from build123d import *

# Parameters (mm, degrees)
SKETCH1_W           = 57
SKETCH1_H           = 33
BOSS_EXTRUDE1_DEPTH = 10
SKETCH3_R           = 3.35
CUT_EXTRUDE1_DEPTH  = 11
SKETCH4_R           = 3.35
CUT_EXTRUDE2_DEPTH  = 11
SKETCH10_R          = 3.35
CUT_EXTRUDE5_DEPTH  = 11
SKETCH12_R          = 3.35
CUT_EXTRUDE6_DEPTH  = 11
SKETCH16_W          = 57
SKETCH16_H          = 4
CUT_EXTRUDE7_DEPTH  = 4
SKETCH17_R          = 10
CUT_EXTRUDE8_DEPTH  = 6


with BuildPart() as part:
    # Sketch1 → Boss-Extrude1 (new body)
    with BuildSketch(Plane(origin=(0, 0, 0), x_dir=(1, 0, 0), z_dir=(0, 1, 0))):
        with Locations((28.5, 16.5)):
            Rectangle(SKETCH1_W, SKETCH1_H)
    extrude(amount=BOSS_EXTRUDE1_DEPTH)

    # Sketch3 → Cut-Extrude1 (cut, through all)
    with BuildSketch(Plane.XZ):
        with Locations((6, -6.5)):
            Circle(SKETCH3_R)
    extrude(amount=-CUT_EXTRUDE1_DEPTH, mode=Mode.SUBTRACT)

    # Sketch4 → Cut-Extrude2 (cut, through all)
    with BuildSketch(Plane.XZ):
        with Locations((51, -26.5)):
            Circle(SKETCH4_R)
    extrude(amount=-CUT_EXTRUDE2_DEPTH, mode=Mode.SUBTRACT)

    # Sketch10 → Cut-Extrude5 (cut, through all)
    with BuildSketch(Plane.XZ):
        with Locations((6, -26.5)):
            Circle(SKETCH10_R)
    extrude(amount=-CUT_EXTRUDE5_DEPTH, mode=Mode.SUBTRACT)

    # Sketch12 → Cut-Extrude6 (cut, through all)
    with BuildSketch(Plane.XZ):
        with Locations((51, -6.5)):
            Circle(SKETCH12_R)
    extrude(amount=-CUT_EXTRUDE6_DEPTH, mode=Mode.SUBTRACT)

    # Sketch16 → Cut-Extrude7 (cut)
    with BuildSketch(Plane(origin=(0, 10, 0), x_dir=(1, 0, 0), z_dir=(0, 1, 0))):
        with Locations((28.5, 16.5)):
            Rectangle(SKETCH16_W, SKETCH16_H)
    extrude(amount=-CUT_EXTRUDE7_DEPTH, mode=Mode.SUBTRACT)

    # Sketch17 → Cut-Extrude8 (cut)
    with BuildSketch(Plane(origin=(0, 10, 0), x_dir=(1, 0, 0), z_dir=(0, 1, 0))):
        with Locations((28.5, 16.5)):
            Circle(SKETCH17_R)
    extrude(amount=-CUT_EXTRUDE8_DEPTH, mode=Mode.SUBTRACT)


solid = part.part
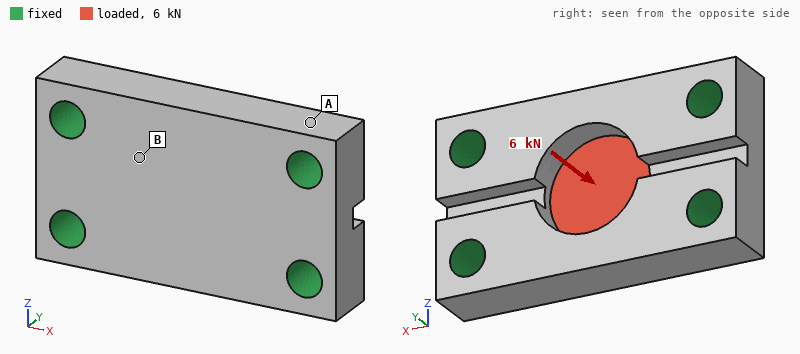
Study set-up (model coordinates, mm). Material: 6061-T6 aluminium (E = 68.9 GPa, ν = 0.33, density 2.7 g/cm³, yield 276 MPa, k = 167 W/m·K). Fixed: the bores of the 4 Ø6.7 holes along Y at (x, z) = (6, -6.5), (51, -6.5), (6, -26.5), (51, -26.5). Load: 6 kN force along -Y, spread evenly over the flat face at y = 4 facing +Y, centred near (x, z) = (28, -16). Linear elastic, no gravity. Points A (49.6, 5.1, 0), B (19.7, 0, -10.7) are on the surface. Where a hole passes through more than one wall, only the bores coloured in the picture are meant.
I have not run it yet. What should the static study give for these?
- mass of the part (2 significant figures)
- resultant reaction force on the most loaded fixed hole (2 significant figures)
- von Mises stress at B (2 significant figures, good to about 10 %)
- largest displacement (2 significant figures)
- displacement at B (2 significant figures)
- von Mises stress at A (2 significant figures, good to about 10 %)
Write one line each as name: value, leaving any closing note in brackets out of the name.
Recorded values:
mass of the part: 40 g
resultant reaction force on the most loaded fixed hole: 1.6 kN
von Mises stress at B: 36 MPa
largest displacement: 40 µm
displacement at B: 18 µm
von Mises stress at A: 14 MPa
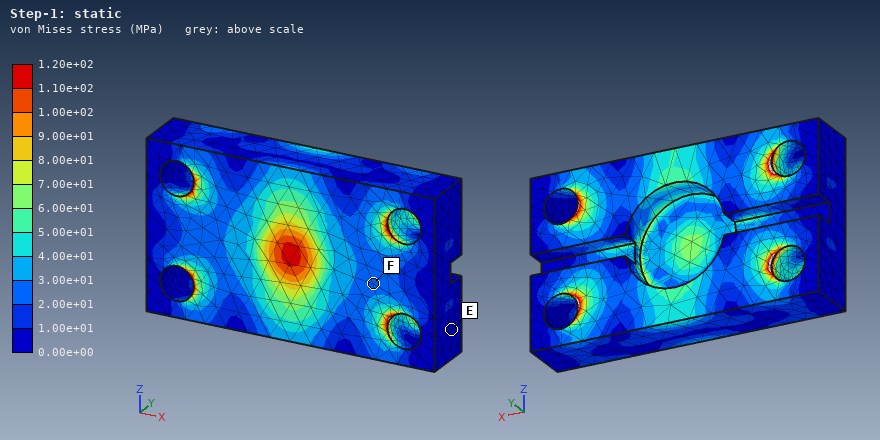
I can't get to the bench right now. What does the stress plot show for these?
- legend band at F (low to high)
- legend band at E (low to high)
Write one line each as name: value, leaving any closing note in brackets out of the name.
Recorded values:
legend band at F: 2.00e+01 to 3.00e+01 MPa
legend band at E: 0.00e+00 to 1.00e+01 MPa
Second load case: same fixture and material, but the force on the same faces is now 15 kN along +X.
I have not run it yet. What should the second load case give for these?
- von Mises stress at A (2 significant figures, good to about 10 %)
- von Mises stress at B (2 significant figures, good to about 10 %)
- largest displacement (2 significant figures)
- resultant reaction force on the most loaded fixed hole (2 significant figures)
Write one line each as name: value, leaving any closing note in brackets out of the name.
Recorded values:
von Mises stress at A: 16 MPa
von Mises stress at B: 46 MPa
largest displacement: 21 µm
resultant reaction force on the most loaded fixed hole: 3.9 kN
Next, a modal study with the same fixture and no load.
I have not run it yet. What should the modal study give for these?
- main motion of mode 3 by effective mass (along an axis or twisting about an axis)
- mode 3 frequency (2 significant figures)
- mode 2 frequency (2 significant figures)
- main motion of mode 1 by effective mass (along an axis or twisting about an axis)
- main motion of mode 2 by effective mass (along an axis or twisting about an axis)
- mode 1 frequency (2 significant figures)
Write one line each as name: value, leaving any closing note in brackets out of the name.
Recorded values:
main motion of mode 3 by effective mass: along Z
mode 3 frequency: 33 kHz
mode 2 frequency: 26 kHz
main motion of mode 1 by effective mass: along Y
main motion of mode 2 by effective mass: twisting about X
mode 1 frequency: 24 kHz
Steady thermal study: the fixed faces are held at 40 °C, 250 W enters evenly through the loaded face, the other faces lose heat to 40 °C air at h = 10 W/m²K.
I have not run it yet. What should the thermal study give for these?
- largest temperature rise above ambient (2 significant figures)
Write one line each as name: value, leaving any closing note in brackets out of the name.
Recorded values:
largest temperature rise above ambient: 77 K
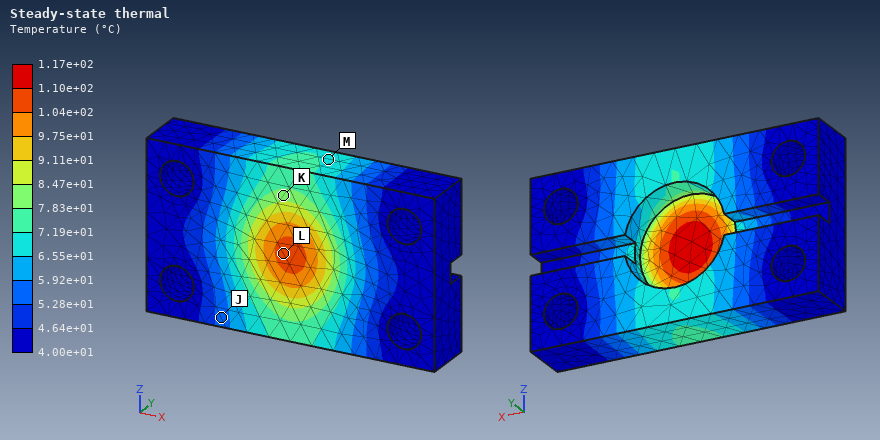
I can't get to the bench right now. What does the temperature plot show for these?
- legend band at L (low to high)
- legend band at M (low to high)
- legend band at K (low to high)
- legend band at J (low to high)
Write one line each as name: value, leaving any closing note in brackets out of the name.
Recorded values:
legend band at L: 1.04e+02 to 1.10e+02 °C
legend band at M: 6.55e+01 to 7.19e+01 °C
legend band at K: 7.83e+01 to 8.47e+01 °C
legend band at J: 5.28e+01 to 5.92e+01 °C
